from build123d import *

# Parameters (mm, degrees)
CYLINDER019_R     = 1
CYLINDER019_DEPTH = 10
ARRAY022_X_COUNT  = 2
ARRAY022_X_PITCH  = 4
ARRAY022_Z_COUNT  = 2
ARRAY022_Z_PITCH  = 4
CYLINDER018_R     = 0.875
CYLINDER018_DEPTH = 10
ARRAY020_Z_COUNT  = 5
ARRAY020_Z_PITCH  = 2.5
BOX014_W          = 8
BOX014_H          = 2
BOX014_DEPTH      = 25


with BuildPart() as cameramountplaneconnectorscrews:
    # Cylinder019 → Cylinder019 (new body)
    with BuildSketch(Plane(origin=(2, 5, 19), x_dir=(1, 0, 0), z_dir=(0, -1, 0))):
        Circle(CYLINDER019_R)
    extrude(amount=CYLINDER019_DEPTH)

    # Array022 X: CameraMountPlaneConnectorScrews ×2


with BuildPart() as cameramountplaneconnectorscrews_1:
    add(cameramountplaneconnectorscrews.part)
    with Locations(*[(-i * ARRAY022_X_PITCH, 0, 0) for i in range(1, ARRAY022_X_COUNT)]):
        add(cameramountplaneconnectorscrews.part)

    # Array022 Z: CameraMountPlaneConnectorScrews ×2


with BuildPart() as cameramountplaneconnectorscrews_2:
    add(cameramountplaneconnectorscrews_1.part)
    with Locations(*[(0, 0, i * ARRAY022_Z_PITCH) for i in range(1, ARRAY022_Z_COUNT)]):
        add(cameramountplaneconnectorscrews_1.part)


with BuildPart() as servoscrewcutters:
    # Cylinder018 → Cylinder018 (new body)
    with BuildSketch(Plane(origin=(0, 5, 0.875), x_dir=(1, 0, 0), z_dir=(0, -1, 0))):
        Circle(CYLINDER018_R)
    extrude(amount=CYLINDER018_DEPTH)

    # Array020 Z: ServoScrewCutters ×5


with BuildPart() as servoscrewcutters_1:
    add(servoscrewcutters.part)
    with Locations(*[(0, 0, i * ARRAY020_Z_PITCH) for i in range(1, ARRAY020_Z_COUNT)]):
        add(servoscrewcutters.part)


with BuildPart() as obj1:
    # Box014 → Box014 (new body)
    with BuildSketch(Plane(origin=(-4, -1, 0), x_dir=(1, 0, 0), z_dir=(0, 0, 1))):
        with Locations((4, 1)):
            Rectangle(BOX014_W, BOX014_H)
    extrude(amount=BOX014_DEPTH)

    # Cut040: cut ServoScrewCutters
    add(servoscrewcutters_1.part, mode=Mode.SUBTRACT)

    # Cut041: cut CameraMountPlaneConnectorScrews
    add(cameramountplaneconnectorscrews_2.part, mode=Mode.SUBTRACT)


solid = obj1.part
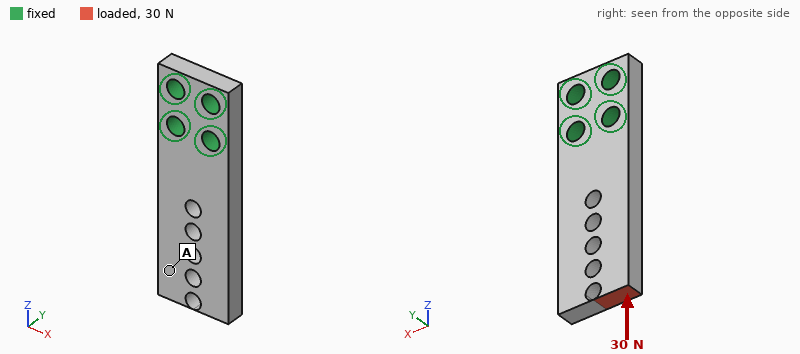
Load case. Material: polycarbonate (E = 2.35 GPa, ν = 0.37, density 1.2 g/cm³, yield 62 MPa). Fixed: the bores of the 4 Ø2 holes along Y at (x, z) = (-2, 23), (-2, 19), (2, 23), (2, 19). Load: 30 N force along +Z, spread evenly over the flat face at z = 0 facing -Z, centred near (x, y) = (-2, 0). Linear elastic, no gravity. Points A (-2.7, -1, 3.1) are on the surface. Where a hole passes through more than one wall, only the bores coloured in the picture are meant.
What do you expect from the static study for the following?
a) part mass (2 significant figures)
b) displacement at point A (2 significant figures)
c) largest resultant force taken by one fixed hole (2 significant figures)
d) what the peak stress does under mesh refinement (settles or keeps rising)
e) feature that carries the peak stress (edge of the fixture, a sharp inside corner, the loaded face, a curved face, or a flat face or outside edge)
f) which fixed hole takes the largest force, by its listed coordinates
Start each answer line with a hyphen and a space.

- 0.42 g
- 0.046 mm
- 25 N
- keeps rising
- a sharp inside corner
- (-2, 19)
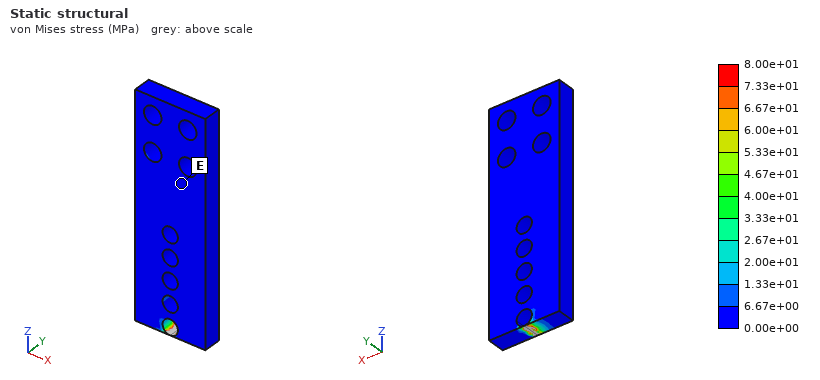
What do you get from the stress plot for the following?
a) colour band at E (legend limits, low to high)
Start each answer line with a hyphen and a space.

- 0.00e+00 to 6.67e+00 MPa
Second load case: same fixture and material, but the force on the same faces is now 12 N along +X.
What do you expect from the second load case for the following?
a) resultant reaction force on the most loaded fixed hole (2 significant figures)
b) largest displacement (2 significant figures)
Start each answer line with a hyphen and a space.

- 40 N
- 0.19 mm
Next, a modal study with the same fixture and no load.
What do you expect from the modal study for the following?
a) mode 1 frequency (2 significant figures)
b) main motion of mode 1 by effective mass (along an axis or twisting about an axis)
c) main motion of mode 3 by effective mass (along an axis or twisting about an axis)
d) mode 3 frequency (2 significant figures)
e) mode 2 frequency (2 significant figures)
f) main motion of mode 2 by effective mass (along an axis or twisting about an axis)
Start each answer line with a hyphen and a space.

- 1400 Hz
- along Y
- twisting about Z
- 5200 Hz
- 4600 Hz
- along X
